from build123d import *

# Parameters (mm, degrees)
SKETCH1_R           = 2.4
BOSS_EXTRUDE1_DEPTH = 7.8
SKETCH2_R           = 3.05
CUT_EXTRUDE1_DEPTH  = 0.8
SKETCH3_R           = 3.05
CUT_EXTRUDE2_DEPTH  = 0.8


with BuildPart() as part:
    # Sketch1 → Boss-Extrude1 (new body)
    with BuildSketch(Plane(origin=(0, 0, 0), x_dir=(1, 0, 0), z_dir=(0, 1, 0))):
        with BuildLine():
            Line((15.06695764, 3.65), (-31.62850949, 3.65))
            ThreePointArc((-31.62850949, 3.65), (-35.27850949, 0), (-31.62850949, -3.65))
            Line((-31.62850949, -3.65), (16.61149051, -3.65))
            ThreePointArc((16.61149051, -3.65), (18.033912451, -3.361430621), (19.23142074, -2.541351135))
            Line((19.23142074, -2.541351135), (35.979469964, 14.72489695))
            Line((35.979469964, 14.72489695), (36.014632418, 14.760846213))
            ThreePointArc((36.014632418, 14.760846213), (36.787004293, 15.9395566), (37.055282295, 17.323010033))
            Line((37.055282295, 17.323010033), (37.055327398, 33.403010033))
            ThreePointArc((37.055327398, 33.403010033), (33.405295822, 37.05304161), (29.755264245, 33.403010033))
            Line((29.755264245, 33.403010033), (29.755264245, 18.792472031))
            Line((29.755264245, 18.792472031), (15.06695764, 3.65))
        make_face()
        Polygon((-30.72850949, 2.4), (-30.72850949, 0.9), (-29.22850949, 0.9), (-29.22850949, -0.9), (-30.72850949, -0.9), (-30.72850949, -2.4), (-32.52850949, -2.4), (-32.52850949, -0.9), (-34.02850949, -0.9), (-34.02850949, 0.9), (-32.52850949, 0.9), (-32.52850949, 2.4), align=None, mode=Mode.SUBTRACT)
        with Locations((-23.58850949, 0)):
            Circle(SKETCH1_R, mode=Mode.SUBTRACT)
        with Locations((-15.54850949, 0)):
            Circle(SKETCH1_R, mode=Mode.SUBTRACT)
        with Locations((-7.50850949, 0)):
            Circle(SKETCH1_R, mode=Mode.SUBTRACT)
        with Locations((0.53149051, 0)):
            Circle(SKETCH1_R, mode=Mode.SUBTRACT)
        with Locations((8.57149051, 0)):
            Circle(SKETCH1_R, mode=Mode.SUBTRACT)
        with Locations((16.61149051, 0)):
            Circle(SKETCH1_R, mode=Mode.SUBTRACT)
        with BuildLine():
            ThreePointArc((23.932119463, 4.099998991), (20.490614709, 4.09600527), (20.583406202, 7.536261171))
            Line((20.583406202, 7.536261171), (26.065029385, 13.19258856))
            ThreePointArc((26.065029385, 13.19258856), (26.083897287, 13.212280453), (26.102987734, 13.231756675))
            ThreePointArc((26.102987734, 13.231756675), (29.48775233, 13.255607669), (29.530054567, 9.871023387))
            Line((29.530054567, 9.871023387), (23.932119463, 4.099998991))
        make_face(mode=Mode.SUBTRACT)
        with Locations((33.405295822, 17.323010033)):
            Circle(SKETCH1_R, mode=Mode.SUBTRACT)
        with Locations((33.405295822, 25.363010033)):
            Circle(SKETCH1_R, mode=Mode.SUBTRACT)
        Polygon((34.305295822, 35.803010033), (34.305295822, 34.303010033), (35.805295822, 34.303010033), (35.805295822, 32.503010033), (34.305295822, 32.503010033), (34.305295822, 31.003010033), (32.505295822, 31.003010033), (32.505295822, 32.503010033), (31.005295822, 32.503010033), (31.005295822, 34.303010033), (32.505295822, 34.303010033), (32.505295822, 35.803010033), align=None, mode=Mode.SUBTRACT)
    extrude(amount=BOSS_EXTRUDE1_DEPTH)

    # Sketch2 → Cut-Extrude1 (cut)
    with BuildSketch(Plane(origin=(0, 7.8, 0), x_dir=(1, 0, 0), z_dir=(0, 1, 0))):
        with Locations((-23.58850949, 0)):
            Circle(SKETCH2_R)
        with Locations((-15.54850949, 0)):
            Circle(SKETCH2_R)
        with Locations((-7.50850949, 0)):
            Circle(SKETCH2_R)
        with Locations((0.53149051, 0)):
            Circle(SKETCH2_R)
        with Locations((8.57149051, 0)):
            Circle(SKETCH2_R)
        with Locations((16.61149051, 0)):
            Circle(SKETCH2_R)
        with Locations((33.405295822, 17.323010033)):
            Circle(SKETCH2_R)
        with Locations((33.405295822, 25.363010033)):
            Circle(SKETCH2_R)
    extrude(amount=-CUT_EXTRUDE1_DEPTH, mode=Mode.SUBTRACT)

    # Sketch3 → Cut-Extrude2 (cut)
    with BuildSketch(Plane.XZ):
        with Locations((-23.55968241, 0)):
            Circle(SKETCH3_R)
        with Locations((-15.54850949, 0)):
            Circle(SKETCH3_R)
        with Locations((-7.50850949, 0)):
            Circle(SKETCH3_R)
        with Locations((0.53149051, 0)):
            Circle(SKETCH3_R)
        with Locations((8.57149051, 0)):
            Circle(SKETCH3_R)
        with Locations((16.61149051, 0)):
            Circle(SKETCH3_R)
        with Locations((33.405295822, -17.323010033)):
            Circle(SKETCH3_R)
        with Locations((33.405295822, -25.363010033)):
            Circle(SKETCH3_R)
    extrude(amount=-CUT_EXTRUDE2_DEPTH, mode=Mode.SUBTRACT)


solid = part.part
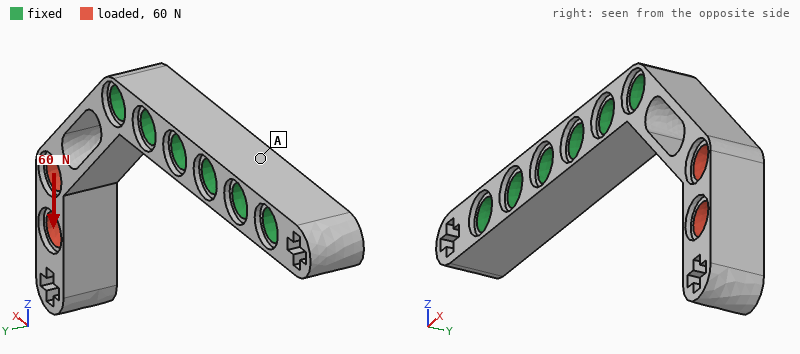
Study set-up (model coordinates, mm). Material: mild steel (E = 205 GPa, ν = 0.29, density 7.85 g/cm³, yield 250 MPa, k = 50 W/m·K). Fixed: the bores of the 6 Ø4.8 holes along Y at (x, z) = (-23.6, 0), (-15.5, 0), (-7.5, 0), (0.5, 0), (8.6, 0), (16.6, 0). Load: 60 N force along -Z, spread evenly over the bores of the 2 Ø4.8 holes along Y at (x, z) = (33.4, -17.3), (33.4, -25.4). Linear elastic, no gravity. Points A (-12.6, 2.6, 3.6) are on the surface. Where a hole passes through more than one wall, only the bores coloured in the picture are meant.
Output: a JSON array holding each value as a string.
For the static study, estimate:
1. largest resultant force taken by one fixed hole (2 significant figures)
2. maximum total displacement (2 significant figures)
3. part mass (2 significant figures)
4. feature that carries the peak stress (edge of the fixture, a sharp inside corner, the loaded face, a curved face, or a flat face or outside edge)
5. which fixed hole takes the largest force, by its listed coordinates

["80 N", "19 µm", "27 g", "a curved face", "(16.6, 0)"]
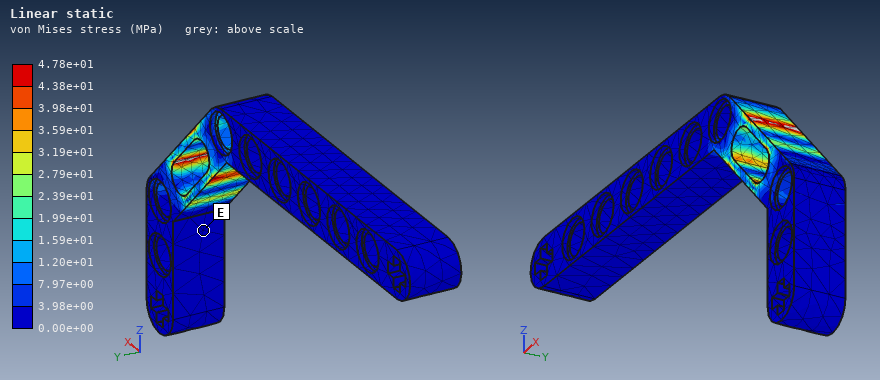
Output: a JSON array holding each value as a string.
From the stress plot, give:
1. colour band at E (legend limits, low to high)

["0.00e+00 to 3.98e+00 MPa"]
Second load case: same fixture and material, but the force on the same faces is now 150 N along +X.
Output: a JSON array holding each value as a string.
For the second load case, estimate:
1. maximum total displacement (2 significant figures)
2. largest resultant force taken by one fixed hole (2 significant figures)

["62 µm", "98 N"]
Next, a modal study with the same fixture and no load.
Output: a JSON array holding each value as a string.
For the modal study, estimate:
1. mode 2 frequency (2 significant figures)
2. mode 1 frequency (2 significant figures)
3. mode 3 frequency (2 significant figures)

["2700 Hz", "2600 Hz", "8300 Hz"]
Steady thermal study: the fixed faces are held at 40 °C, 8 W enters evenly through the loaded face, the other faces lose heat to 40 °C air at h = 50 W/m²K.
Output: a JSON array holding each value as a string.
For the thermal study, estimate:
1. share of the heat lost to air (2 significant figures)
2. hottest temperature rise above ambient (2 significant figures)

["52 %", "80 K"]
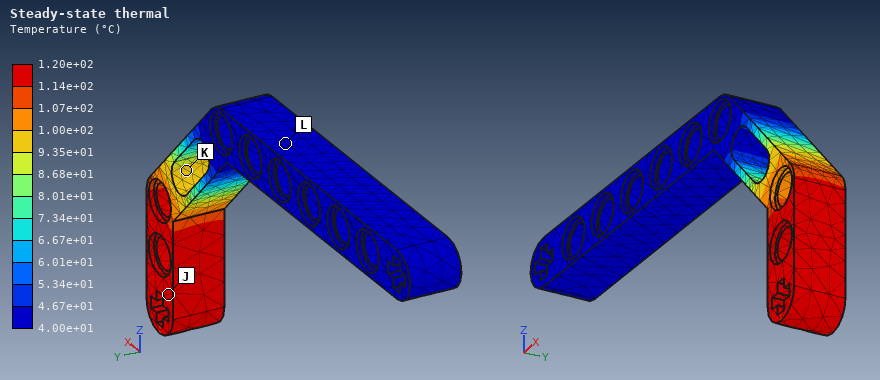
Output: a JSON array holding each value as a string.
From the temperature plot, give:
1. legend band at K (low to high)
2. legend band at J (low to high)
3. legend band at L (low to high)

["9.35e+01 to 1.00e+02 °C", "1.14e+02 to 1.20e+02 °C", "4.00e+01 to 4.67e+01 °C"]
